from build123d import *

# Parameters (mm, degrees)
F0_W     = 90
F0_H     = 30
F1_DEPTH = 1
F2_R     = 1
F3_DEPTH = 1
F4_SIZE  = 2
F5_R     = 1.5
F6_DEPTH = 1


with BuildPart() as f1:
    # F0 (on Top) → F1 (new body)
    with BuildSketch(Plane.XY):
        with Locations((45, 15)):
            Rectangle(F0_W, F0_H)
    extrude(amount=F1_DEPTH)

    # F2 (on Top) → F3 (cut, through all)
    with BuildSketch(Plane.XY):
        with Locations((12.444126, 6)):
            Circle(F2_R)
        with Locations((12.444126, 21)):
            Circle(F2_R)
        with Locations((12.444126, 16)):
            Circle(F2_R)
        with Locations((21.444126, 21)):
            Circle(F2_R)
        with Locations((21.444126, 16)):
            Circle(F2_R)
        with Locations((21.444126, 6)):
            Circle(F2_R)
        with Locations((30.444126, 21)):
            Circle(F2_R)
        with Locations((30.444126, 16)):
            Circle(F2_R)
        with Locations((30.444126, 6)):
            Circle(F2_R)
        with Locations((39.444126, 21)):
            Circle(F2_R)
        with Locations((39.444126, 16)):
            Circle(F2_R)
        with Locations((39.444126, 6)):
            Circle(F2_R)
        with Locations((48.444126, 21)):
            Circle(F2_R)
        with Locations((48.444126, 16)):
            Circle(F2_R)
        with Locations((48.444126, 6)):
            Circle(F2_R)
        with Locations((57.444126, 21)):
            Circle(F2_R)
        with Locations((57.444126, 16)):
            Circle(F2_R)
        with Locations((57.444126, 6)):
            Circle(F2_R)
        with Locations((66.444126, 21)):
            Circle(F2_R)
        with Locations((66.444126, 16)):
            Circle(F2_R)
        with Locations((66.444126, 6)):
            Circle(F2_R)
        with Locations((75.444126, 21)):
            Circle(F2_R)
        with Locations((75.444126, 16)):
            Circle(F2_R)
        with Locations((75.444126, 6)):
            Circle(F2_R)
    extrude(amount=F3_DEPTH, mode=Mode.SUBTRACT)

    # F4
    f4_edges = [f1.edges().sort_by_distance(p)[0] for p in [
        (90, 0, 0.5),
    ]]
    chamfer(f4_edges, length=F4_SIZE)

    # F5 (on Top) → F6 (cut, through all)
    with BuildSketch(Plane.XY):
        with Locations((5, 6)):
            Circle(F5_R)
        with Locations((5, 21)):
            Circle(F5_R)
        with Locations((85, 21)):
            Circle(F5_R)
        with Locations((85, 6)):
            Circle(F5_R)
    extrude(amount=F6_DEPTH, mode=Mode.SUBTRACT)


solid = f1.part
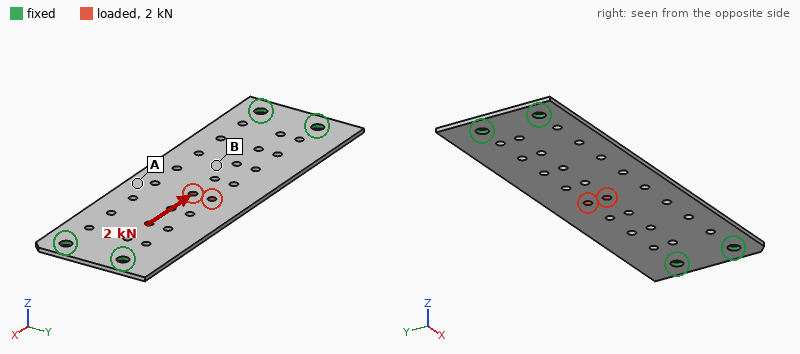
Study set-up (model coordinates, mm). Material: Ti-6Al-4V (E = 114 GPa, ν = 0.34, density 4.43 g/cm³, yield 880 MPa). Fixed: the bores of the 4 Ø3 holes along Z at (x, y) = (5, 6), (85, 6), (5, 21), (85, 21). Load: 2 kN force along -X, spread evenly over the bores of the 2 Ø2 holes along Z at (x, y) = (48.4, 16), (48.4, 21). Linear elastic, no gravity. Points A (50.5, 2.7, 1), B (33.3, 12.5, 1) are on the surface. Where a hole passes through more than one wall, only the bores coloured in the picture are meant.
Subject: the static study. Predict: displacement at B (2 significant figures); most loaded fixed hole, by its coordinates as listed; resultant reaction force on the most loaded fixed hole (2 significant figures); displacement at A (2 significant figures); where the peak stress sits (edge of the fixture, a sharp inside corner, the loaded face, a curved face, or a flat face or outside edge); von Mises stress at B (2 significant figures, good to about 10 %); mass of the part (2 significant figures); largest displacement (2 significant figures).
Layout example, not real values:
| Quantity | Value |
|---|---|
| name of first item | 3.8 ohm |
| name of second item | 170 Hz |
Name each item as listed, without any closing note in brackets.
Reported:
| Quantity | Value |
|---|---|
| displacement at B | 9.8 µm |
| most loaded fixed hole, by its coordinates as listed | (85, 21) |
| resultant reaction force on the most loaded fixed hole | 610 N |
| displacement at A | 8.2 µm |
| where the peak stress sits | the loaded face |
| von Mises stress at B | 45 MPa |
| mass of the part | 11 g |
| largest displacement | 21 µm |
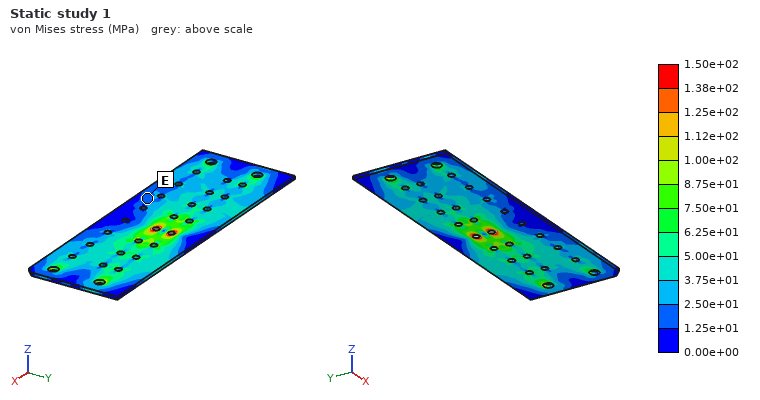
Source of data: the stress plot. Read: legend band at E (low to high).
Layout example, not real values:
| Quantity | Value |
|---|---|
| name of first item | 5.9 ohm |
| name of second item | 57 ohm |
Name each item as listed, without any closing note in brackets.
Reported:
| Quantity | Value |
|---|---|
| legend band at E | 1.25e+01 to 2.50e+01 MPa |
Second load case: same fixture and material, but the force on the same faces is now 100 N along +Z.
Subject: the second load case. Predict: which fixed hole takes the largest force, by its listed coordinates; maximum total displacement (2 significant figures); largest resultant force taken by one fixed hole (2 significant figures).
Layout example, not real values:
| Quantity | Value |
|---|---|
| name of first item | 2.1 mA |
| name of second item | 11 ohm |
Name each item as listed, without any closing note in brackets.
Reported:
| Quantity | Value |
|---|---|
| which fixed hole takes the largest force, by its listed coordinates | (85, 21) |
| maximum total displacement | 1.1 mm |
| largest resultant force taken by one fixed hole | 42 N |
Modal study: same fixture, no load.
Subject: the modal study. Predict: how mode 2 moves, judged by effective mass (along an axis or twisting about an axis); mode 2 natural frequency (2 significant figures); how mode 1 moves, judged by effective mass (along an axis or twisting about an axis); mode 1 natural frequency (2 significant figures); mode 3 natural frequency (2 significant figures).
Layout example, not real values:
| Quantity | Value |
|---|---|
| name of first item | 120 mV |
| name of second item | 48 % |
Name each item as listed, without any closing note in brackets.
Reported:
| Quantity | Value |
|---|---|
| how mode 2 moves, judged by effective mass | twisting about X |
| mode 2 natural frequency | 1600 Hz |
| how mode 1 moves, judged by effective mass | along Z |
| mode 1 natural frequency | 840 Hz |
| mode 3 natural frequency | 2300 Hz |
